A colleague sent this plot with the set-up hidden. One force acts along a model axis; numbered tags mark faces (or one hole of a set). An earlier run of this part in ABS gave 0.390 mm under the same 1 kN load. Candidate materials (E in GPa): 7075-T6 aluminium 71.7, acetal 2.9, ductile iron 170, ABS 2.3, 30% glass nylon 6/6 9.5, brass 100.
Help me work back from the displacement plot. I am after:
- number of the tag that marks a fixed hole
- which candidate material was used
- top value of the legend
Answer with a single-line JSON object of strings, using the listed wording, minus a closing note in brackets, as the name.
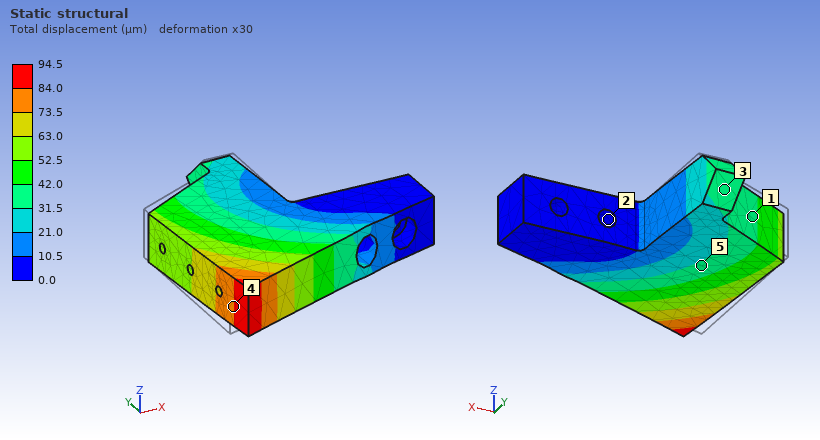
{"number of the tag that marks a fixed hole": "2", "which candidate material was used": "30% glass nylon 6/6", "top value of the legend": "94.5 µm"}
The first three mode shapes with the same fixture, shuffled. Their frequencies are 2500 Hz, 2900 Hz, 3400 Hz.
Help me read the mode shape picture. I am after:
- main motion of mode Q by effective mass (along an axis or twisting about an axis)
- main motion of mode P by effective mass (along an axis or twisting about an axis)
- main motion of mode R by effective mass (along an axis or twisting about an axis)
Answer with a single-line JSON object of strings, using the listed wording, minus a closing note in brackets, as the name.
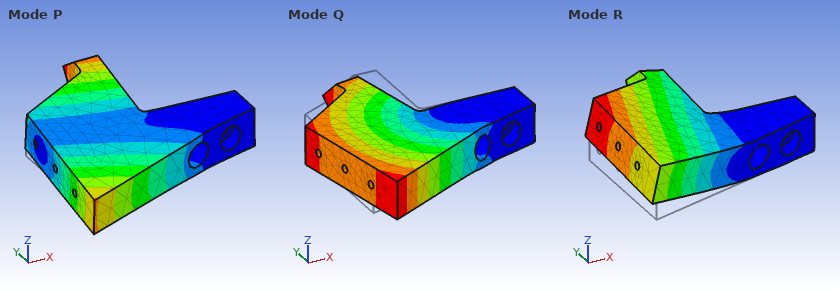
{"main motion of mode Q by effective mass": "along Y", "main motion of mode P by effective mass": "twisting about X", "main motion of mode R by effective mass": "along Z"}
